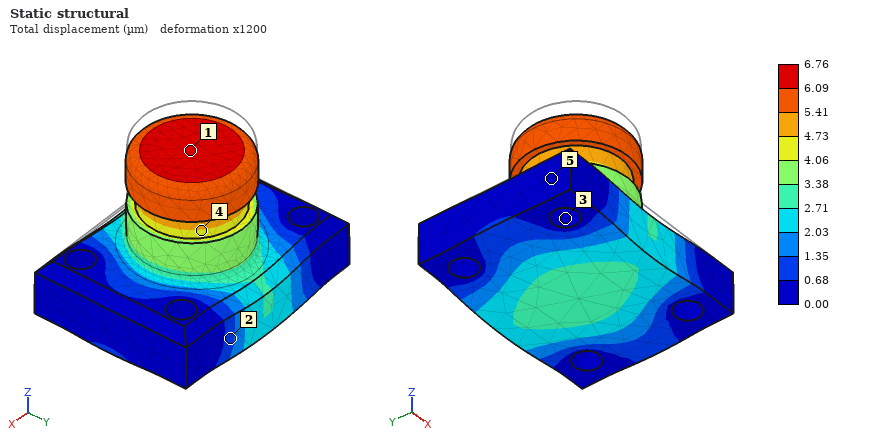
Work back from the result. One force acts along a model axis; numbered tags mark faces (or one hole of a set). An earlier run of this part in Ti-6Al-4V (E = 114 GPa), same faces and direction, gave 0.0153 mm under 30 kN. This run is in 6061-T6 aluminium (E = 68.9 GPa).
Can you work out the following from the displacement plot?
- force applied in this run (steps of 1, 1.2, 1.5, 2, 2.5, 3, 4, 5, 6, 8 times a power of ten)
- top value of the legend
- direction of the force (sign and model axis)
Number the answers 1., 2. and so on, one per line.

1. 8 kN
2. 6.76 µm
3. -Z
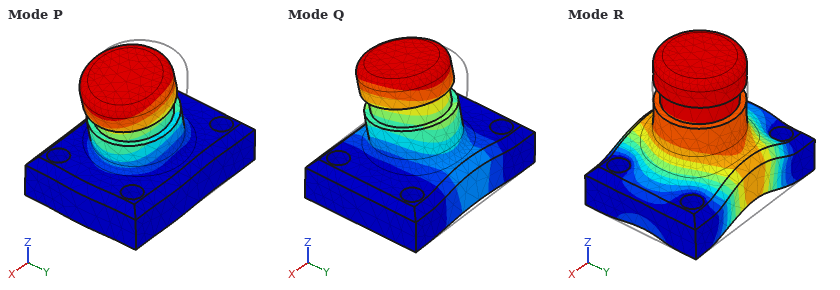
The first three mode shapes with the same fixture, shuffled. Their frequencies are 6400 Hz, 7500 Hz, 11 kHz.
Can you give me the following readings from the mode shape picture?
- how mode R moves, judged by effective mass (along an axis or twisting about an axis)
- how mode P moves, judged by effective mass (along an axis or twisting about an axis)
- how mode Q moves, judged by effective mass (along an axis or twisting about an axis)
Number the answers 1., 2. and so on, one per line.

1. along Z
2. along X
3. along Y
